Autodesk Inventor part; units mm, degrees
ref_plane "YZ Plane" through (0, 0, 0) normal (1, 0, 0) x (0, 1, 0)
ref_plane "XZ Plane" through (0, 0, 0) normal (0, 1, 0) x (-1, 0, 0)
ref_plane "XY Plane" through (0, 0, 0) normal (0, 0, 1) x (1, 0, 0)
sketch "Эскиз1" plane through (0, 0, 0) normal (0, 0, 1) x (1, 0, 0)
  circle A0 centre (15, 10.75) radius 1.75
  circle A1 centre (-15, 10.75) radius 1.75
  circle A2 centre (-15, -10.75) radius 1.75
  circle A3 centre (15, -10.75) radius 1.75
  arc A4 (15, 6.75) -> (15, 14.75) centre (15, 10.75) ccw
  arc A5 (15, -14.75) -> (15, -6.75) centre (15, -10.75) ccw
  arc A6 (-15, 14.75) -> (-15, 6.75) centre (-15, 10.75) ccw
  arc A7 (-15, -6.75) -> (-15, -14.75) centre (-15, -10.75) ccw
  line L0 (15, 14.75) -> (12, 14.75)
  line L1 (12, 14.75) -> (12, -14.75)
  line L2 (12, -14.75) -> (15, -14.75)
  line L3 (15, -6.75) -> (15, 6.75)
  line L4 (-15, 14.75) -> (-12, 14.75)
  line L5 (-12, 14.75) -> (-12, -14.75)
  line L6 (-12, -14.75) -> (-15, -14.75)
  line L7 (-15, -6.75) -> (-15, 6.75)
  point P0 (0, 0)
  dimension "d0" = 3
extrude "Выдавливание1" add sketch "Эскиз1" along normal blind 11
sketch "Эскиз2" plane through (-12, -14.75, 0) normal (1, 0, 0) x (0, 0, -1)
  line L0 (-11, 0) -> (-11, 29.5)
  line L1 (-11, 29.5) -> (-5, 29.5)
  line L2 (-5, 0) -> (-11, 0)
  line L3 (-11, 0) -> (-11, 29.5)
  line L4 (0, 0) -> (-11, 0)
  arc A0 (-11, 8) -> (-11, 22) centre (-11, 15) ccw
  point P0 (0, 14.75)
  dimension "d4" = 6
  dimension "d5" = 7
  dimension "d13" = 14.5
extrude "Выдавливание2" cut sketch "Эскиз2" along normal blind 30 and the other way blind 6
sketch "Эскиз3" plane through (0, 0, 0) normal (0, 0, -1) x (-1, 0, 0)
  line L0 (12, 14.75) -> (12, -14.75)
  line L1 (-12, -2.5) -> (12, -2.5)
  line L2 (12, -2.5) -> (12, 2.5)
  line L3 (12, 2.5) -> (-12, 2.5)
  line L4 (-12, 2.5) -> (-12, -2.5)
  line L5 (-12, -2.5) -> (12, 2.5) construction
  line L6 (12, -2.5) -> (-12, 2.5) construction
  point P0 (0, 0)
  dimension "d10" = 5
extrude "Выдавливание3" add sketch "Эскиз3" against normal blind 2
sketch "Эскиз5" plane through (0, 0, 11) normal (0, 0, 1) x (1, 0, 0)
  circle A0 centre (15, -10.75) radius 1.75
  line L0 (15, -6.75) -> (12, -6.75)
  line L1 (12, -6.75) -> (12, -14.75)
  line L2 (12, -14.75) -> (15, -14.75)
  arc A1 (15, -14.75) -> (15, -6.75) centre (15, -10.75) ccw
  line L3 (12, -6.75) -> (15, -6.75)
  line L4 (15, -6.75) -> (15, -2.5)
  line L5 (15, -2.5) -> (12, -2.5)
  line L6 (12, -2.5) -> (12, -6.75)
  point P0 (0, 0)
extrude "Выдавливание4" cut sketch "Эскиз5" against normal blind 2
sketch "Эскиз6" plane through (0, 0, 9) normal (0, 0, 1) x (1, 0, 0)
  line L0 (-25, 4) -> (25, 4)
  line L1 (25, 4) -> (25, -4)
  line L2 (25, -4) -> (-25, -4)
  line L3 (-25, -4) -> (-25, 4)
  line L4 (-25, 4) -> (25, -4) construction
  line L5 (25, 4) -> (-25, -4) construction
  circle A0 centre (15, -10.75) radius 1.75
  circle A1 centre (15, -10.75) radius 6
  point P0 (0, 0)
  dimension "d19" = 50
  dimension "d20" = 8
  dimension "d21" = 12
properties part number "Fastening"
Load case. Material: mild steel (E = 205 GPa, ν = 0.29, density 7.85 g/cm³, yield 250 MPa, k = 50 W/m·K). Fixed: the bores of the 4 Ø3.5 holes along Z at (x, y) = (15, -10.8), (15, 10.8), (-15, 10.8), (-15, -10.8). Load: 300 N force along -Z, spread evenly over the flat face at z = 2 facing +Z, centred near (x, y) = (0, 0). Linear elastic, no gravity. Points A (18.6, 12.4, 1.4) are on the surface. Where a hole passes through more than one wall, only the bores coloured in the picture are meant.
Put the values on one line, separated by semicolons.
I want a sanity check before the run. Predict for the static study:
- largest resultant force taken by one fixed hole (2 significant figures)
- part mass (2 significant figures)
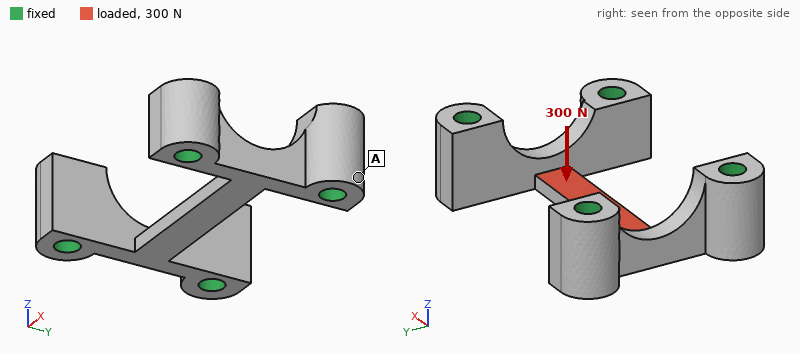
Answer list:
100 N; 18 g
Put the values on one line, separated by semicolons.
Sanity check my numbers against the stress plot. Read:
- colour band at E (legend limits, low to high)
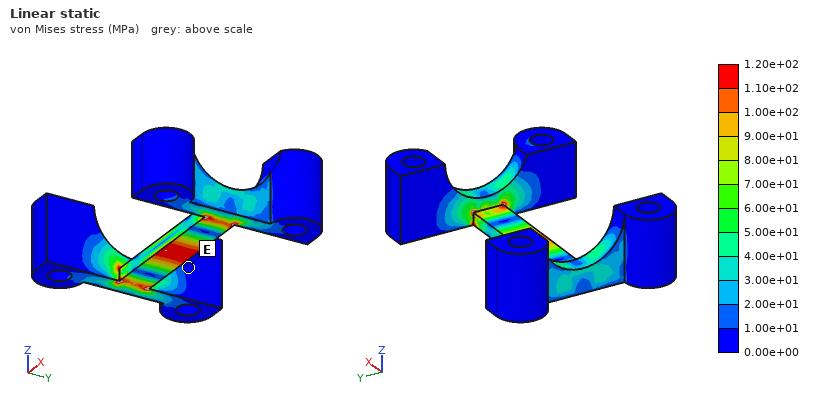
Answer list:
0.00e+00 to 1.00e+01 MPa
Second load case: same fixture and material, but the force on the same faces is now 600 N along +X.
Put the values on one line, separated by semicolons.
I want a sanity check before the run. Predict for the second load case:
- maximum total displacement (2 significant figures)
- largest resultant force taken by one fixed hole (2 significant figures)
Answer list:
4.7 µm; 170 N
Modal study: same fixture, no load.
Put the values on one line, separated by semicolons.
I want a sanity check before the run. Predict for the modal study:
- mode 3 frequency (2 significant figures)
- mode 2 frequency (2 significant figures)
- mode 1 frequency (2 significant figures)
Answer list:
33 kHz; 28 kHz; 14 kHz
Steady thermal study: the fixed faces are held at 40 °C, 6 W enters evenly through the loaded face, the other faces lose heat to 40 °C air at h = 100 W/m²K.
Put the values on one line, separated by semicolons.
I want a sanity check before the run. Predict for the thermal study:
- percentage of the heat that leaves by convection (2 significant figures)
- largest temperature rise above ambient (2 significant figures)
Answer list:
18 %; 47 K
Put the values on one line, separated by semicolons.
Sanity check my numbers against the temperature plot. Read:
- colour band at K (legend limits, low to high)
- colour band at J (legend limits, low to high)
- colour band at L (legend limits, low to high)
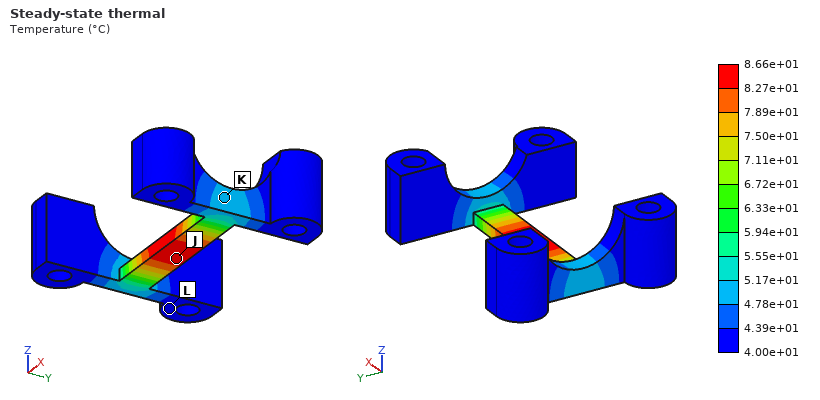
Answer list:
4.78e+01 to 5.17e+01 °C; 8.27e+01 to 8.66e+01 °C; 4.00e+01 to 4.39e+01 °C
